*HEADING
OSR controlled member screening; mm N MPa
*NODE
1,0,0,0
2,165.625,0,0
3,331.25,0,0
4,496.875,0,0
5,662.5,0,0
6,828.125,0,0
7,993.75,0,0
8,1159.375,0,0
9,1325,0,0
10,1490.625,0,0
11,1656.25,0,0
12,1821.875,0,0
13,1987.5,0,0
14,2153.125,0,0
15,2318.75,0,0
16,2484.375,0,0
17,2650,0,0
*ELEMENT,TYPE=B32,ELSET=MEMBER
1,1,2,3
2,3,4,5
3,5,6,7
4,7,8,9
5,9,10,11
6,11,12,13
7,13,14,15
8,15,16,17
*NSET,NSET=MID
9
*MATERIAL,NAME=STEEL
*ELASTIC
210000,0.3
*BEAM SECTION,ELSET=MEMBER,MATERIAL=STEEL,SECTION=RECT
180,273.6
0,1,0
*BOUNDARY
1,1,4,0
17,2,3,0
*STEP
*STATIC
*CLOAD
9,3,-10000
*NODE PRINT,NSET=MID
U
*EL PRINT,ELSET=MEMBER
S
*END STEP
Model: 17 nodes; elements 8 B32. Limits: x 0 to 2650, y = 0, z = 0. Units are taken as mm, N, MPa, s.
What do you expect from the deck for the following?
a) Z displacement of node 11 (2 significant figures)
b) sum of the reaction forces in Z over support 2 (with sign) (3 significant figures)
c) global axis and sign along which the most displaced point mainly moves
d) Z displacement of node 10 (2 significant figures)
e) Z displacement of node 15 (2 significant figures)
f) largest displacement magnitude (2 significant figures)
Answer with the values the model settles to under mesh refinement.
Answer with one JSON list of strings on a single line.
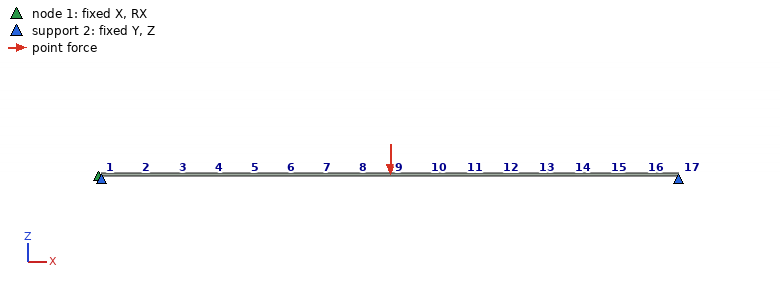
["-0.056 mm", "10000 N", "-Z", "-0.060 mm", "-0.023 mm", "0.062 mm"]
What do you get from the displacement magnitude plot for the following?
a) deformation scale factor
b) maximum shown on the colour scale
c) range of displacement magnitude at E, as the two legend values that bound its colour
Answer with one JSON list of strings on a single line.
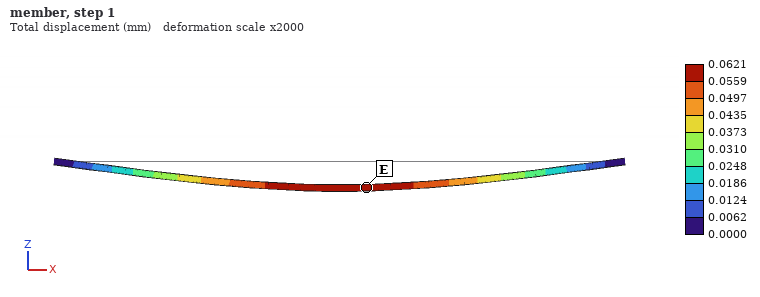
["2000", "0.0621 mm", "0.0559 to 0.0621 mm"]
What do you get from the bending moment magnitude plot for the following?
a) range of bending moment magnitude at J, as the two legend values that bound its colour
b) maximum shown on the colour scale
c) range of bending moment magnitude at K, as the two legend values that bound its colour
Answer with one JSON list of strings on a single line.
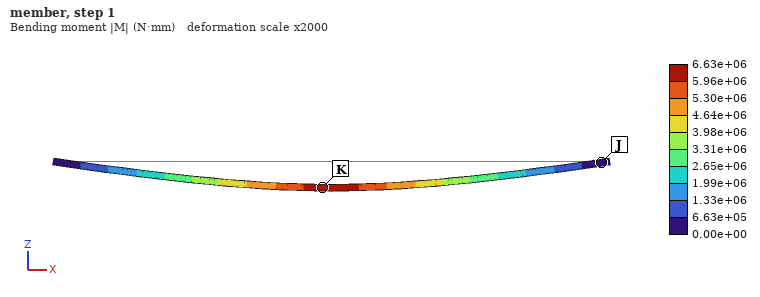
["0.00e+00 to 6.63e+05 N·mm", "6.63e+06 N·mm", "5.96e+06 to 6.63e+06 N·mm"]
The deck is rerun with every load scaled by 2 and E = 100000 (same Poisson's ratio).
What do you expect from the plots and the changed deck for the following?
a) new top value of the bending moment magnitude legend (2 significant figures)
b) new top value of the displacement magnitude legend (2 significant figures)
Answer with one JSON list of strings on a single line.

["1.3e+07 N·mm", "0.26 mm"]
